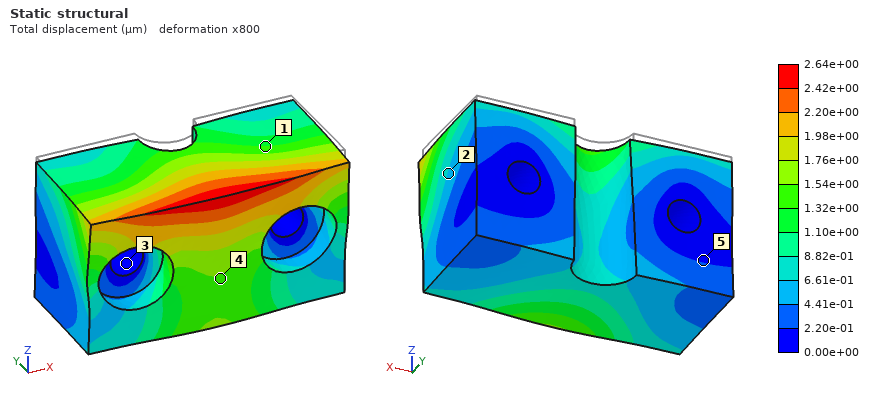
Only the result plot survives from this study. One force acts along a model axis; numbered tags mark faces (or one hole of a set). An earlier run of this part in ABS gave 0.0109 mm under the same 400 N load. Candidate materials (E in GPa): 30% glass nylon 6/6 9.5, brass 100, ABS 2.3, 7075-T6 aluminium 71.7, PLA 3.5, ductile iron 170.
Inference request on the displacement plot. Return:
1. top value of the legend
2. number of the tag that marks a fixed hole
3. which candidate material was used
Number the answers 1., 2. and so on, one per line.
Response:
1. 2.64e+00 µm
2. 3
3. 30% glass nylon 6/6
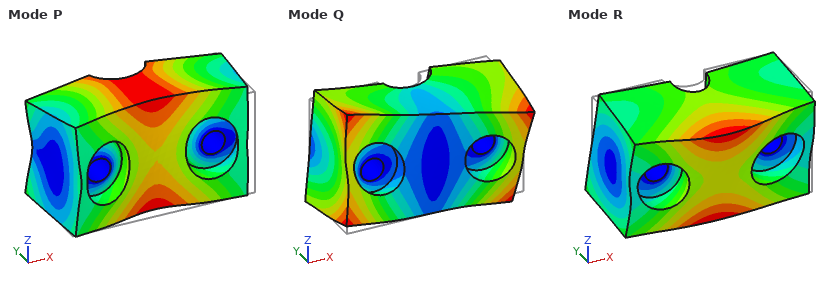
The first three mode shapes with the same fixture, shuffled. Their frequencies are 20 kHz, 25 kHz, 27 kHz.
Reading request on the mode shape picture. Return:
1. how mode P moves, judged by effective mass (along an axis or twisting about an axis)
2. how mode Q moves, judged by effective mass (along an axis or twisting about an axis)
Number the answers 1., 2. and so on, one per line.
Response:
1. along Y
2. twisting about Y
